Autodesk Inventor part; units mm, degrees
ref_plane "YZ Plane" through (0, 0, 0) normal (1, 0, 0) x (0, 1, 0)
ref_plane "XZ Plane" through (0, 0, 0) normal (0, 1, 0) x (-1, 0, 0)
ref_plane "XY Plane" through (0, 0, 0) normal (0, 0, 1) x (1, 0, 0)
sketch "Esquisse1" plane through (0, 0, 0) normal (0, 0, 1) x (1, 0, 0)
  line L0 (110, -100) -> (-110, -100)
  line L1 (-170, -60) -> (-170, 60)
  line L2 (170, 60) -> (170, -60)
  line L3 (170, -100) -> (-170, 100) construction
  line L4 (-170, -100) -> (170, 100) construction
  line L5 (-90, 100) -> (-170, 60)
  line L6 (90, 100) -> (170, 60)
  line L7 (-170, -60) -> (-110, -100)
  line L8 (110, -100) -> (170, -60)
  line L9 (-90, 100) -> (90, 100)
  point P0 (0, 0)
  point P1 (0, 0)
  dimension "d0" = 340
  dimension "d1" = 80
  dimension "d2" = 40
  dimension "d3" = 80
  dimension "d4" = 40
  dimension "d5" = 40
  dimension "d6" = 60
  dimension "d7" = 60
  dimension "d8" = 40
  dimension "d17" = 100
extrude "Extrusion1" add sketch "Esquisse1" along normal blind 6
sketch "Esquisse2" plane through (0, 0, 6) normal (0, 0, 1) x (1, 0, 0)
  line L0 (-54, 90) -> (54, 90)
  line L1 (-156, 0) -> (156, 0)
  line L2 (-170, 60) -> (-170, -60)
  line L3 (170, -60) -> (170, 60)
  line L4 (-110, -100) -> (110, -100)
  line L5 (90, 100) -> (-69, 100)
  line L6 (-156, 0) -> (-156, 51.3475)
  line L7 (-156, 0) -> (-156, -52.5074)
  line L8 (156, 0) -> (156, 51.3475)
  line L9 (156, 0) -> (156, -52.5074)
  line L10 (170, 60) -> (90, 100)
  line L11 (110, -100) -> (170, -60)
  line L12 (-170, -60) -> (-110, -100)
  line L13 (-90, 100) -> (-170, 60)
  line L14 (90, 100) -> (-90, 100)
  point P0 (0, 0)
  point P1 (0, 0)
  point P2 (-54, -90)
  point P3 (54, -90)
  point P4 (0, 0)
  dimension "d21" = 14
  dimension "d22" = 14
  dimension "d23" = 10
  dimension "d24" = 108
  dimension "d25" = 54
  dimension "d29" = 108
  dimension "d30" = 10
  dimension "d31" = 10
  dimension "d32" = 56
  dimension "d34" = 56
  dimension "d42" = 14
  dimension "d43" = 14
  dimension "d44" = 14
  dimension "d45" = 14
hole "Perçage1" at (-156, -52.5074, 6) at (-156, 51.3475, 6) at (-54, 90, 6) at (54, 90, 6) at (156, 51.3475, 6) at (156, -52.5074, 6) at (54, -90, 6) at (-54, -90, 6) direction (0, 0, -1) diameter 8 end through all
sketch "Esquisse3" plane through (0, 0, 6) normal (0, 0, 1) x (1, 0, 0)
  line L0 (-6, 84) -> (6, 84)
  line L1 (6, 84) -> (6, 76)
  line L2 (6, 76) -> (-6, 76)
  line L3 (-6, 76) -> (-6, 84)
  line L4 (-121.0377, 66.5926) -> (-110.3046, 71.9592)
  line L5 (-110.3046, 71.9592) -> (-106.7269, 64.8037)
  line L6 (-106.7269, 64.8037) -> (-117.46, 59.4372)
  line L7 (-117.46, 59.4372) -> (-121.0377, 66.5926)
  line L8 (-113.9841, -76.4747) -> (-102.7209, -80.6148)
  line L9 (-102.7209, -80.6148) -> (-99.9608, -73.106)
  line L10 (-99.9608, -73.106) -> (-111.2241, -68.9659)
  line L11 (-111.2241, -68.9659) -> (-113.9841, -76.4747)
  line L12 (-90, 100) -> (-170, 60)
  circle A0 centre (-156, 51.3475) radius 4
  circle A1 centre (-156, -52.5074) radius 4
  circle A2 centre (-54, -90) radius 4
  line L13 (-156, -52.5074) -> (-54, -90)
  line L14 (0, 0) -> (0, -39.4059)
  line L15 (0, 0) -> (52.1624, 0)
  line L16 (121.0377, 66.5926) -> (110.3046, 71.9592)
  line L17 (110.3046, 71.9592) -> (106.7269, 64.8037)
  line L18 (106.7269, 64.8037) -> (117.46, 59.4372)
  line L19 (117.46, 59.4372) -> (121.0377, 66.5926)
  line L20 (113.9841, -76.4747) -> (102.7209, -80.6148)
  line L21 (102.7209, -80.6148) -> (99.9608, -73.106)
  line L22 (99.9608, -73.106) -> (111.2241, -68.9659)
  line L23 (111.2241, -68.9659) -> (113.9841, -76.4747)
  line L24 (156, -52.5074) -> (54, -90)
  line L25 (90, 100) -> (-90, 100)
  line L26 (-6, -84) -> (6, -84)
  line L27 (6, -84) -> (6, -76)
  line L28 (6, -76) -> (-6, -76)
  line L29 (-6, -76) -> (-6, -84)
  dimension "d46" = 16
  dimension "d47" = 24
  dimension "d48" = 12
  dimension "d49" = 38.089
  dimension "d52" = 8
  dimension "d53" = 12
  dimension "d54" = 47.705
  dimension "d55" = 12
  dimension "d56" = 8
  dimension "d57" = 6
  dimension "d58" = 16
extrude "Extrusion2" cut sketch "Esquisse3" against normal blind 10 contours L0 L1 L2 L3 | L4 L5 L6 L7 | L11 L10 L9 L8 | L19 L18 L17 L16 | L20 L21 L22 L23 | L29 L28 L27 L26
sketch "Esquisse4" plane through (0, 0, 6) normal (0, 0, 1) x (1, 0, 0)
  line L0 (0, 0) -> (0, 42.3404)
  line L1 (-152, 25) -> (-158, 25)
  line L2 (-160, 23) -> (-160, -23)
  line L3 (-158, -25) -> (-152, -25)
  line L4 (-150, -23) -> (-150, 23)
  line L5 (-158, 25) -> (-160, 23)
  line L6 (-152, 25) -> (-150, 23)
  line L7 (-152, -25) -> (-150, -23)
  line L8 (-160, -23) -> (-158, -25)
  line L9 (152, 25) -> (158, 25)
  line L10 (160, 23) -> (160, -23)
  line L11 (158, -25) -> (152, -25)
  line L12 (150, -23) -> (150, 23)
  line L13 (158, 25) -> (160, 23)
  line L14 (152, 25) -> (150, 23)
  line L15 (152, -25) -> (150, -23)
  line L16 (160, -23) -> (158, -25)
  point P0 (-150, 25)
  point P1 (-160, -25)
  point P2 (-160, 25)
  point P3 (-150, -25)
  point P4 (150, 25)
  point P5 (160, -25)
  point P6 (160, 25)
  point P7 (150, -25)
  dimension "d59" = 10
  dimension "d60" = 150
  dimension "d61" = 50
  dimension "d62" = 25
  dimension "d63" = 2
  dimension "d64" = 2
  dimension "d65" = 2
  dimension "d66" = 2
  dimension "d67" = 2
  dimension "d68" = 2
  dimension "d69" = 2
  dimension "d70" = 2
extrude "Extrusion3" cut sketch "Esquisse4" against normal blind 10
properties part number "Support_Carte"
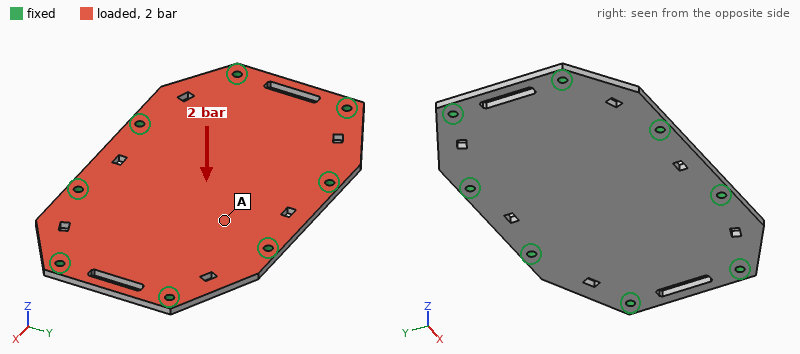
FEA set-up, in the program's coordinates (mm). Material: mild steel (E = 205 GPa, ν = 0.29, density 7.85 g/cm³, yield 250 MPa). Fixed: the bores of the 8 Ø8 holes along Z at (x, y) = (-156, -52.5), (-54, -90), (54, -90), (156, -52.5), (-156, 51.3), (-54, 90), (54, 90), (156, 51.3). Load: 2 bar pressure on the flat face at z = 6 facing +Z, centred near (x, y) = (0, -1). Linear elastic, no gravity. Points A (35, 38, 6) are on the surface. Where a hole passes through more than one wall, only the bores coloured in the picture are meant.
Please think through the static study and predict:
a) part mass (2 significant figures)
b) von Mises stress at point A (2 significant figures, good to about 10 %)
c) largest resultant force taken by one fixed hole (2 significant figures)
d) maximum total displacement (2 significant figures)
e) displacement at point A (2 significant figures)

2.8 kg
27 MPa
2.0 kN
0.20 mm
0.14 mm
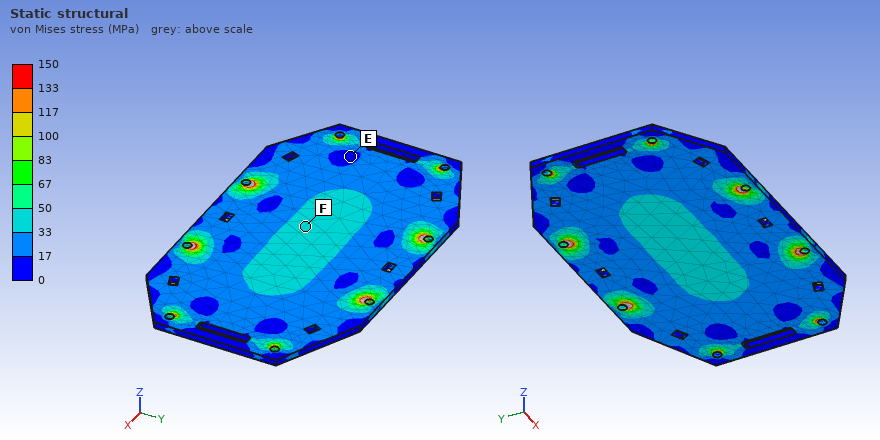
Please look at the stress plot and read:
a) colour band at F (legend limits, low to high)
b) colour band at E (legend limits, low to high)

33 to 50 MPa
0 to 17 MPa
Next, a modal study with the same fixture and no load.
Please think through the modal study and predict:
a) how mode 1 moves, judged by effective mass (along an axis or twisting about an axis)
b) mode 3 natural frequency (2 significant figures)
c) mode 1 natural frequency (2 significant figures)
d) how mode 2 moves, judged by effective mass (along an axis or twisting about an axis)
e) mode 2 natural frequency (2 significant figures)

along Z
1800 Hz
910 Hz
twisting about Y
1300 Hz
